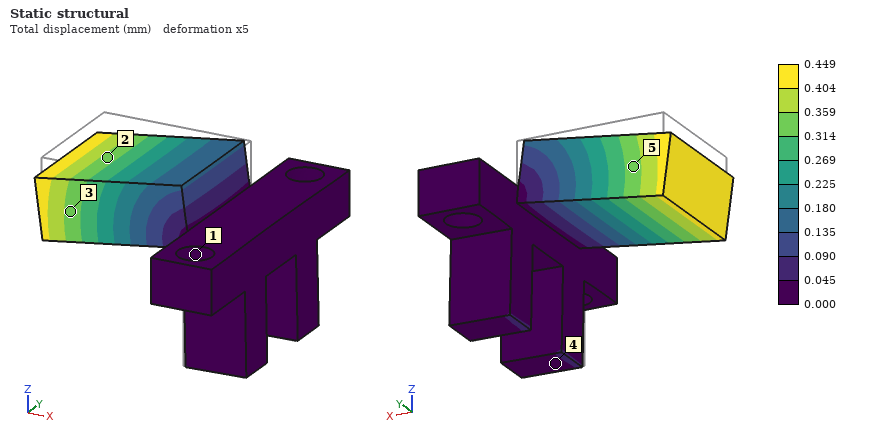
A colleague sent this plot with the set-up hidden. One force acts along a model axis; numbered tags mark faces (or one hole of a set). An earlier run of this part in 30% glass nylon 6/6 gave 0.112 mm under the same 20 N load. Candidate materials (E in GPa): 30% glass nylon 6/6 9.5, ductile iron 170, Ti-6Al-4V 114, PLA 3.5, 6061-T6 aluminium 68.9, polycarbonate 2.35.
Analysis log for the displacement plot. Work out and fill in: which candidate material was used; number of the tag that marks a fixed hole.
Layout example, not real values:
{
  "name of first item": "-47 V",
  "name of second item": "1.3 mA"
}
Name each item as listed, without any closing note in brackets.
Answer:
{
  "which candidate material was used": "polycarbonate",
  "number of the tag that marks a fixed hole": "1"
}
